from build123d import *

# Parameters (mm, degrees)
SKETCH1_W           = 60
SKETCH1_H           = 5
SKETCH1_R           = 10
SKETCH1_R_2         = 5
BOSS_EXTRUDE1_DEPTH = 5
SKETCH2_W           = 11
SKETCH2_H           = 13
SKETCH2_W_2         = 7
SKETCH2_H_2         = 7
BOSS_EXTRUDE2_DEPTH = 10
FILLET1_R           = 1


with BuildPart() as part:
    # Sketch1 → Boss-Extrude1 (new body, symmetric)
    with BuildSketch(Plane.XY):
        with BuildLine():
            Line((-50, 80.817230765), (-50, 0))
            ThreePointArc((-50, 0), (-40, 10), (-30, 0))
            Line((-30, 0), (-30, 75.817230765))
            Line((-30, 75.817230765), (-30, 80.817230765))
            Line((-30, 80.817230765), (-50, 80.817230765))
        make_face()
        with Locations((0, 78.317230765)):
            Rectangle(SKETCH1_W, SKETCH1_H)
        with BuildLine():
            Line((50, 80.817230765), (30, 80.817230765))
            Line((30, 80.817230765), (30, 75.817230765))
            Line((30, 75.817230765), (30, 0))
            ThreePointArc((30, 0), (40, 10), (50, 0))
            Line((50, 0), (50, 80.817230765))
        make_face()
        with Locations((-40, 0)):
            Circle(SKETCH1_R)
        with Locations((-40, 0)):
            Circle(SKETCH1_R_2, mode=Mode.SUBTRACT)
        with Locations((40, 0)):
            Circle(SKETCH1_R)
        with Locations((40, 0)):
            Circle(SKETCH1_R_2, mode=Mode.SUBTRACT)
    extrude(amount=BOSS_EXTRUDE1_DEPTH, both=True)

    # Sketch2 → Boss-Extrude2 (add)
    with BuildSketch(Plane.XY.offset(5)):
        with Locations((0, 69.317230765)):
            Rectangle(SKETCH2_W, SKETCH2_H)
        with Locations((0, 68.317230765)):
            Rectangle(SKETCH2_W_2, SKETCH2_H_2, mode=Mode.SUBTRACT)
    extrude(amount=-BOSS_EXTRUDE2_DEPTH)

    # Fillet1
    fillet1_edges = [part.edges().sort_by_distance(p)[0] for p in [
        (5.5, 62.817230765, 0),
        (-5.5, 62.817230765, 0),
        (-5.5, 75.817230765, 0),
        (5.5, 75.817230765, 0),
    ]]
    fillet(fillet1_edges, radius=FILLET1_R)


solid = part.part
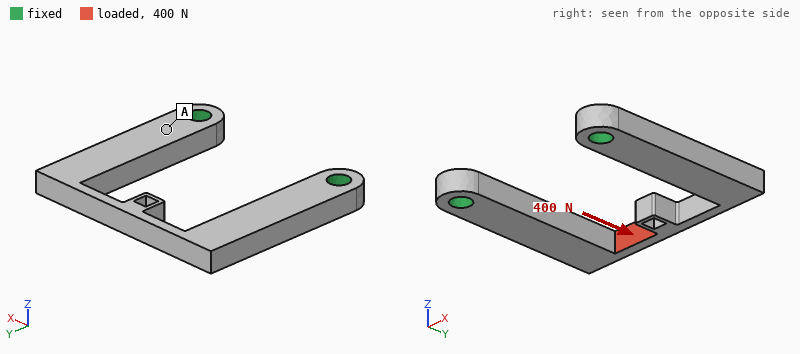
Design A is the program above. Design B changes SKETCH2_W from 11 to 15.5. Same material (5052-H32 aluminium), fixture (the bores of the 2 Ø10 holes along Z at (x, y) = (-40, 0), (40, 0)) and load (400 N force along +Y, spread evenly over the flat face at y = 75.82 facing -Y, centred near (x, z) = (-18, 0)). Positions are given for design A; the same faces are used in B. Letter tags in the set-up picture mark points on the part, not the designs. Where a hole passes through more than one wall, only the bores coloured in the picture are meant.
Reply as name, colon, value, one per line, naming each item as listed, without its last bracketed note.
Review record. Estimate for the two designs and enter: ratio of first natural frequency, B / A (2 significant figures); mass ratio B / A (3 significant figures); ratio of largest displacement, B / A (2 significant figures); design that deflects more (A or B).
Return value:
ratio of first natural frequency, B / A: 0.98
mass ratio B / A: 1.02
ratio of largest displacement, B / A: 0.92
design that deflects more: A
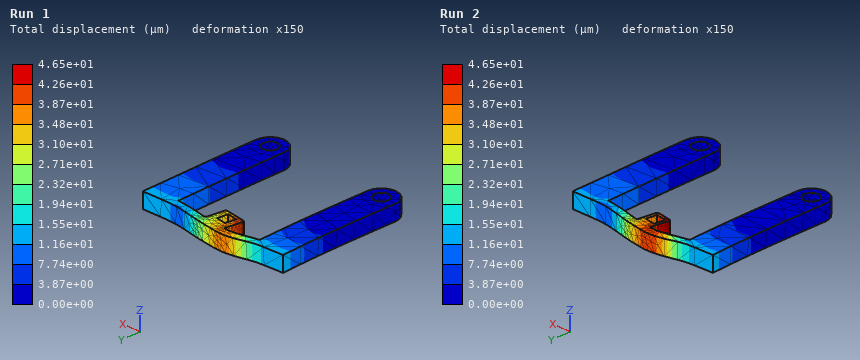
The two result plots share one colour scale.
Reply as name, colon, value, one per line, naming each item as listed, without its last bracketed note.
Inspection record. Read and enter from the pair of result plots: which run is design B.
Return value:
which run is design B: Run 1
